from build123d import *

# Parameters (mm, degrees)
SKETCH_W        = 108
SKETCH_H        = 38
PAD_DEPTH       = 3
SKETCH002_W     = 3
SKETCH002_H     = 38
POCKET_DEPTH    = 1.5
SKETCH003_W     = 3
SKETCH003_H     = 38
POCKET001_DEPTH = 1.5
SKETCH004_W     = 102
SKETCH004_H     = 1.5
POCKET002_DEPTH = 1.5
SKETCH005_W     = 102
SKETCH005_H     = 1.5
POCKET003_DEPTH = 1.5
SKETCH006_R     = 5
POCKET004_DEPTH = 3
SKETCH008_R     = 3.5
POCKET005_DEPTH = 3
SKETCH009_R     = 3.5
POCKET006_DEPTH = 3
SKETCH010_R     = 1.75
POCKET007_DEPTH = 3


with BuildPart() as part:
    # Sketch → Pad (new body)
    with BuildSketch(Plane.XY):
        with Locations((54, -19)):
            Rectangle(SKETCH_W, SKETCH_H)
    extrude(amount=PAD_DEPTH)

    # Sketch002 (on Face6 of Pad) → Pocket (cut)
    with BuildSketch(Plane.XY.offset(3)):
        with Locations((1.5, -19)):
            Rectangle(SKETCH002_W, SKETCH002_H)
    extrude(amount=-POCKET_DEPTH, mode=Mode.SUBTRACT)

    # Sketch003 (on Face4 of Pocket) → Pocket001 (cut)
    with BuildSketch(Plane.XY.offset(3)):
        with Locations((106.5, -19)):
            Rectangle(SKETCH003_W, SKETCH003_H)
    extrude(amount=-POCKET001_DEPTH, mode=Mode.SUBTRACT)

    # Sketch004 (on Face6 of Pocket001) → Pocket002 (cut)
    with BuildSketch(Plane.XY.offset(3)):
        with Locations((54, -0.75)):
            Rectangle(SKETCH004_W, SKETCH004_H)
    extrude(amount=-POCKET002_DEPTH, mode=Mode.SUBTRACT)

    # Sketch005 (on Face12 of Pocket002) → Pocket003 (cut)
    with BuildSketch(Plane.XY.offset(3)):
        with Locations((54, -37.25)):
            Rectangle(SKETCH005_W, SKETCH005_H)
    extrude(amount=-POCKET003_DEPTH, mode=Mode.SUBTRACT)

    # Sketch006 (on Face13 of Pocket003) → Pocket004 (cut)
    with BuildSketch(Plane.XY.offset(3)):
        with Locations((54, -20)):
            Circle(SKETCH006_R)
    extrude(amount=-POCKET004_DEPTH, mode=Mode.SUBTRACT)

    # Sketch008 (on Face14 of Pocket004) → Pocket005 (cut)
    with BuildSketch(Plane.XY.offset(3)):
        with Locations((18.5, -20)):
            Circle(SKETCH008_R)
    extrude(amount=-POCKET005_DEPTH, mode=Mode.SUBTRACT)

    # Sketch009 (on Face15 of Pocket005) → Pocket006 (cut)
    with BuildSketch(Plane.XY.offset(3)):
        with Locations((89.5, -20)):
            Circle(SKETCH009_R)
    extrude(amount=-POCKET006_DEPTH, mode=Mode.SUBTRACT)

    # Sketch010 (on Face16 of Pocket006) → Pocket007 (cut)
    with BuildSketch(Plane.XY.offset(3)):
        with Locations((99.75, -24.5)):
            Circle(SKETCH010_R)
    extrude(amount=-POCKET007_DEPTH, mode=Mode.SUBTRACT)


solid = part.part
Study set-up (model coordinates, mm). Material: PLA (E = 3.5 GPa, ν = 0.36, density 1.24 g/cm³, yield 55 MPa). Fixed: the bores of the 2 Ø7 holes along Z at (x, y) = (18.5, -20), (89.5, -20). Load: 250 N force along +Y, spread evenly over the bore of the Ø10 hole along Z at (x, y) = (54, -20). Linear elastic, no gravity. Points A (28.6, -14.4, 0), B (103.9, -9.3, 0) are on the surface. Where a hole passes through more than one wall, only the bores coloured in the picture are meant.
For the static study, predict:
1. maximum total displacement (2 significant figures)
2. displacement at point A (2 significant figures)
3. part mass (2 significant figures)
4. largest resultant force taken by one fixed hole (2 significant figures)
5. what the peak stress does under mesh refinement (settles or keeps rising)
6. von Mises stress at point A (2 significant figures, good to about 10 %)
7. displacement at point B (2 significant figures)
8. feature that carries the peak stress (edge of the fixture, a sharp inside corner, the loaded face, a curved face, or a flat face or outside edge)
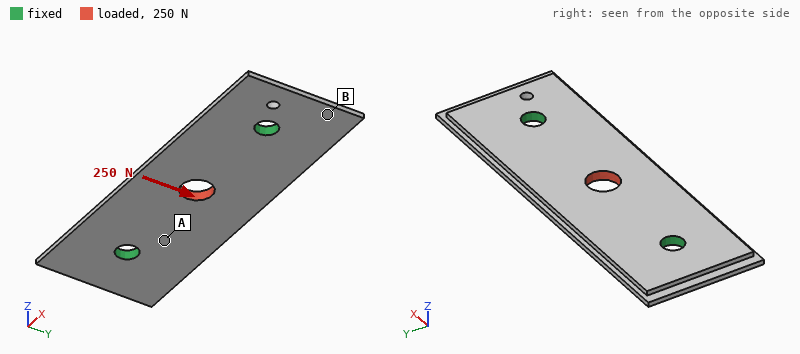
67 µm
22 µm
14 g
130 N
keeps rising
2.9 MPa
19 µm
edge of the fixture
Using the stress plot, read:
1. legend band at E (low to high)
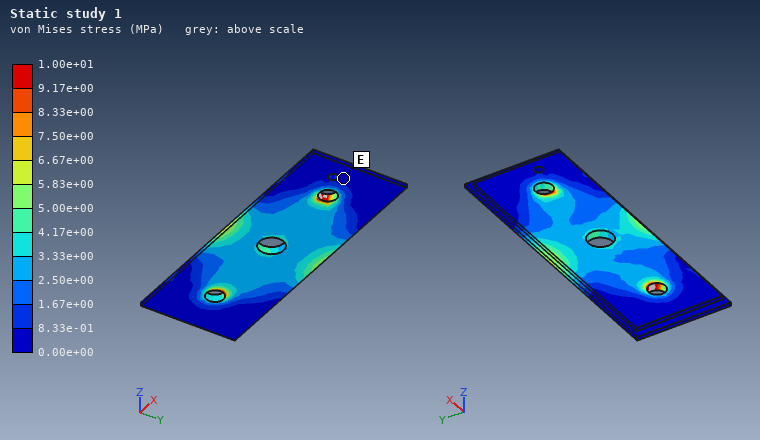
0.00e+00 to 8.33e-01 MPa
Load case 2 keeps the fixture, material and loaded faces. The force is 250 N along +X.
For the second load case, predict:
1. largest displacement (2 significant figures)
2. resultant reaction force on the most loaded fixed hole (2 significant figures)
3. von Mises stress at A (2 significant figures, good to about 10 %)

19 µm
130 N
1.6 MPa
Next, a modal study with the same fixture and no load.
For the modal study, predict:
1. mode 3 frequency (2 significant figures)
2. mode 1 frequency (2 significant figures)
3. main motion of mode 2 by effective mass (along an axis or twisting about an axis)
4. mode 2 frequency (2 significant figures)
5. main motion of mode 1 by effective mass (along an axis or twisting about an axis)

2300 Hz
1000 Hz
twisting about X
1300 Hz
along Z
